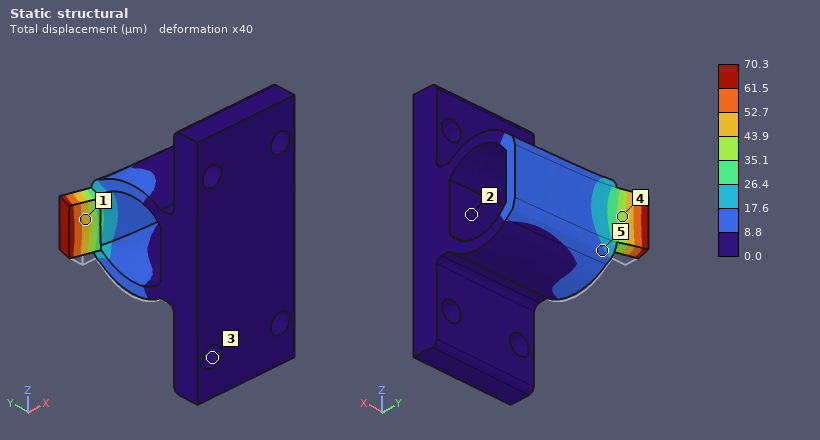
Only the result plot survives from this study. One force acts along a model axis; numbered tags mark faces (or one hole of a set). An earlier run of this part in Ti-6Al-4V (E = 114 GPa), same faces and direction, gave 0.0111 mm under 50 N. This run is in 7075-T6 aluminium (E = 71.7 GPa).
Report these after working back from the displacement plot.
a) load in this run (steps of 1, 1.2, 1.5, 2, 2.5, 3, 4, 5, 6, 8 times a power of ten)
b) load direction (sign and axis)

200 N
+Y
